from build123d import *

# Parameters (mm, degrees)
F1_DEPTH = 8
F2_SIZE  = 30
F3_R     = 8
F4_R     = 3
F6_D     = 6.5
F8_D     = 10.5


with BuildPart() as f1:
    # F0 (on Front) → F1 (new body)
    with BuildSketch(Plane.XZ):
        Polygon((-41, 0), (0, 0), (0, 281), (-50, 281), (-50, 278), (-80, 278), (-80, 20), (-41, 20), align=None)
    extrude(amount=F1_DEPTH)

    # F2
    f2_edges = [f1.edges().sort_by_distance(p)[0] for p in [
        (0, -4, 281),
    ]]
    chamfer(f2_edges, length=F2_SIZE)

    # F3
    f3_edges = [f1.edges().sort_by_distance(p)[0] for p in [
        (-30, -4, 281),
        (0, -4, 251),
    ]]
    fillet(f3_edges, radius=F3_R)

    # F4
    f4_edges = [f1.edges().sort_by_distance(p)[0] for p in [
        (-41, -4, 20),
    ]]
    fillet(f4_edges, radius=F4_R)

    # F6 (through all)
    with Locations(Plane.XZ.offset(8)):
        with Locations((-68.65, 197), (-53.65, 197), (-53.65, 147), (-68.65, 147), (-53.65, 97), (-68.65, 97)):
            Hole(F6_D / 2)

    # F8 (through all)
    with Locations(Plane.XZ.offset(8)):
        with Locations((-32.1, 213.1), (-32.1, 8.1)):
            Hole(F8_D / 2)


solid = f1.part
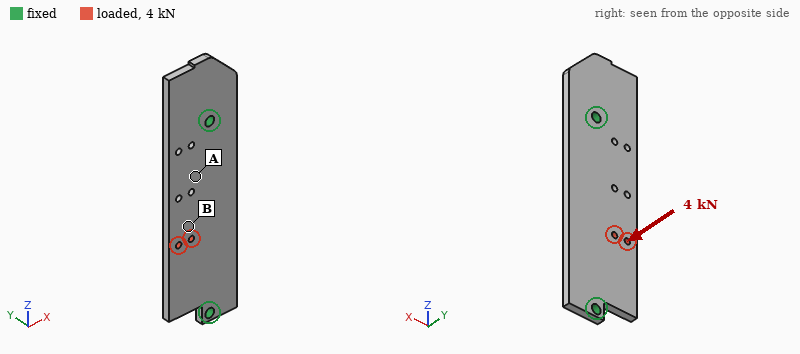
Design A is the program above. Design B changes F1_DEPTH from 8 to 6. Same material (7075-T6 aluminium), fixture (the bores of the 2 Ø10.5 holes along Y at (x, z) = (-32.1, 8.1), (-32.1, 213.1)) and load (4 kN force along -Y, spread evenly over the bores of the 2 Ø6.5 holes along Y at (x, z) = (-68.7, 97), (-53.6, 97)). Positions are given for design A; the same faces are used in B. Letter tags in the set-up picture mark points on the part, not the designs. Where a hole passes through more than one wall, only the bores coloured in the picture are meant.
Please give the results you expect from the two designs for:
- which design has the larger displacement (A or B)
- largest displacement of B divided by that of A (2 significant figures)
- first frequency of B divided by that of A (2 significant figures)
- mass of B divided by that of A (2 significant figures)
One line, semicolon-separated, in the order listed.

B; 2.3; 0.76; 0.75
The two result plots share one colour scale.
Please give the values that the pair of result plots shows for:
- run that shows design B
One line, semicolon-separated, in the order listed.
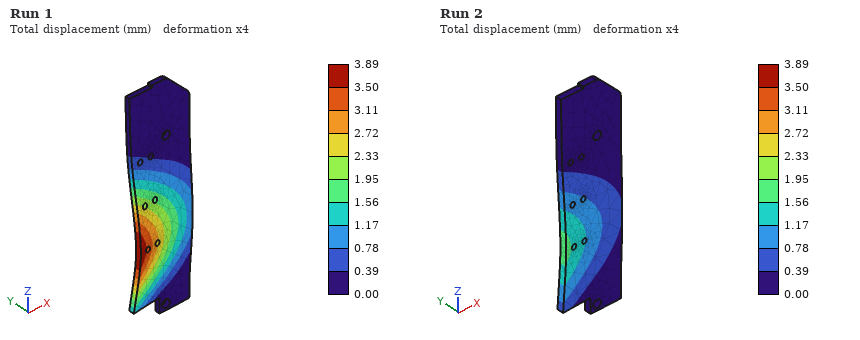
Run 1
